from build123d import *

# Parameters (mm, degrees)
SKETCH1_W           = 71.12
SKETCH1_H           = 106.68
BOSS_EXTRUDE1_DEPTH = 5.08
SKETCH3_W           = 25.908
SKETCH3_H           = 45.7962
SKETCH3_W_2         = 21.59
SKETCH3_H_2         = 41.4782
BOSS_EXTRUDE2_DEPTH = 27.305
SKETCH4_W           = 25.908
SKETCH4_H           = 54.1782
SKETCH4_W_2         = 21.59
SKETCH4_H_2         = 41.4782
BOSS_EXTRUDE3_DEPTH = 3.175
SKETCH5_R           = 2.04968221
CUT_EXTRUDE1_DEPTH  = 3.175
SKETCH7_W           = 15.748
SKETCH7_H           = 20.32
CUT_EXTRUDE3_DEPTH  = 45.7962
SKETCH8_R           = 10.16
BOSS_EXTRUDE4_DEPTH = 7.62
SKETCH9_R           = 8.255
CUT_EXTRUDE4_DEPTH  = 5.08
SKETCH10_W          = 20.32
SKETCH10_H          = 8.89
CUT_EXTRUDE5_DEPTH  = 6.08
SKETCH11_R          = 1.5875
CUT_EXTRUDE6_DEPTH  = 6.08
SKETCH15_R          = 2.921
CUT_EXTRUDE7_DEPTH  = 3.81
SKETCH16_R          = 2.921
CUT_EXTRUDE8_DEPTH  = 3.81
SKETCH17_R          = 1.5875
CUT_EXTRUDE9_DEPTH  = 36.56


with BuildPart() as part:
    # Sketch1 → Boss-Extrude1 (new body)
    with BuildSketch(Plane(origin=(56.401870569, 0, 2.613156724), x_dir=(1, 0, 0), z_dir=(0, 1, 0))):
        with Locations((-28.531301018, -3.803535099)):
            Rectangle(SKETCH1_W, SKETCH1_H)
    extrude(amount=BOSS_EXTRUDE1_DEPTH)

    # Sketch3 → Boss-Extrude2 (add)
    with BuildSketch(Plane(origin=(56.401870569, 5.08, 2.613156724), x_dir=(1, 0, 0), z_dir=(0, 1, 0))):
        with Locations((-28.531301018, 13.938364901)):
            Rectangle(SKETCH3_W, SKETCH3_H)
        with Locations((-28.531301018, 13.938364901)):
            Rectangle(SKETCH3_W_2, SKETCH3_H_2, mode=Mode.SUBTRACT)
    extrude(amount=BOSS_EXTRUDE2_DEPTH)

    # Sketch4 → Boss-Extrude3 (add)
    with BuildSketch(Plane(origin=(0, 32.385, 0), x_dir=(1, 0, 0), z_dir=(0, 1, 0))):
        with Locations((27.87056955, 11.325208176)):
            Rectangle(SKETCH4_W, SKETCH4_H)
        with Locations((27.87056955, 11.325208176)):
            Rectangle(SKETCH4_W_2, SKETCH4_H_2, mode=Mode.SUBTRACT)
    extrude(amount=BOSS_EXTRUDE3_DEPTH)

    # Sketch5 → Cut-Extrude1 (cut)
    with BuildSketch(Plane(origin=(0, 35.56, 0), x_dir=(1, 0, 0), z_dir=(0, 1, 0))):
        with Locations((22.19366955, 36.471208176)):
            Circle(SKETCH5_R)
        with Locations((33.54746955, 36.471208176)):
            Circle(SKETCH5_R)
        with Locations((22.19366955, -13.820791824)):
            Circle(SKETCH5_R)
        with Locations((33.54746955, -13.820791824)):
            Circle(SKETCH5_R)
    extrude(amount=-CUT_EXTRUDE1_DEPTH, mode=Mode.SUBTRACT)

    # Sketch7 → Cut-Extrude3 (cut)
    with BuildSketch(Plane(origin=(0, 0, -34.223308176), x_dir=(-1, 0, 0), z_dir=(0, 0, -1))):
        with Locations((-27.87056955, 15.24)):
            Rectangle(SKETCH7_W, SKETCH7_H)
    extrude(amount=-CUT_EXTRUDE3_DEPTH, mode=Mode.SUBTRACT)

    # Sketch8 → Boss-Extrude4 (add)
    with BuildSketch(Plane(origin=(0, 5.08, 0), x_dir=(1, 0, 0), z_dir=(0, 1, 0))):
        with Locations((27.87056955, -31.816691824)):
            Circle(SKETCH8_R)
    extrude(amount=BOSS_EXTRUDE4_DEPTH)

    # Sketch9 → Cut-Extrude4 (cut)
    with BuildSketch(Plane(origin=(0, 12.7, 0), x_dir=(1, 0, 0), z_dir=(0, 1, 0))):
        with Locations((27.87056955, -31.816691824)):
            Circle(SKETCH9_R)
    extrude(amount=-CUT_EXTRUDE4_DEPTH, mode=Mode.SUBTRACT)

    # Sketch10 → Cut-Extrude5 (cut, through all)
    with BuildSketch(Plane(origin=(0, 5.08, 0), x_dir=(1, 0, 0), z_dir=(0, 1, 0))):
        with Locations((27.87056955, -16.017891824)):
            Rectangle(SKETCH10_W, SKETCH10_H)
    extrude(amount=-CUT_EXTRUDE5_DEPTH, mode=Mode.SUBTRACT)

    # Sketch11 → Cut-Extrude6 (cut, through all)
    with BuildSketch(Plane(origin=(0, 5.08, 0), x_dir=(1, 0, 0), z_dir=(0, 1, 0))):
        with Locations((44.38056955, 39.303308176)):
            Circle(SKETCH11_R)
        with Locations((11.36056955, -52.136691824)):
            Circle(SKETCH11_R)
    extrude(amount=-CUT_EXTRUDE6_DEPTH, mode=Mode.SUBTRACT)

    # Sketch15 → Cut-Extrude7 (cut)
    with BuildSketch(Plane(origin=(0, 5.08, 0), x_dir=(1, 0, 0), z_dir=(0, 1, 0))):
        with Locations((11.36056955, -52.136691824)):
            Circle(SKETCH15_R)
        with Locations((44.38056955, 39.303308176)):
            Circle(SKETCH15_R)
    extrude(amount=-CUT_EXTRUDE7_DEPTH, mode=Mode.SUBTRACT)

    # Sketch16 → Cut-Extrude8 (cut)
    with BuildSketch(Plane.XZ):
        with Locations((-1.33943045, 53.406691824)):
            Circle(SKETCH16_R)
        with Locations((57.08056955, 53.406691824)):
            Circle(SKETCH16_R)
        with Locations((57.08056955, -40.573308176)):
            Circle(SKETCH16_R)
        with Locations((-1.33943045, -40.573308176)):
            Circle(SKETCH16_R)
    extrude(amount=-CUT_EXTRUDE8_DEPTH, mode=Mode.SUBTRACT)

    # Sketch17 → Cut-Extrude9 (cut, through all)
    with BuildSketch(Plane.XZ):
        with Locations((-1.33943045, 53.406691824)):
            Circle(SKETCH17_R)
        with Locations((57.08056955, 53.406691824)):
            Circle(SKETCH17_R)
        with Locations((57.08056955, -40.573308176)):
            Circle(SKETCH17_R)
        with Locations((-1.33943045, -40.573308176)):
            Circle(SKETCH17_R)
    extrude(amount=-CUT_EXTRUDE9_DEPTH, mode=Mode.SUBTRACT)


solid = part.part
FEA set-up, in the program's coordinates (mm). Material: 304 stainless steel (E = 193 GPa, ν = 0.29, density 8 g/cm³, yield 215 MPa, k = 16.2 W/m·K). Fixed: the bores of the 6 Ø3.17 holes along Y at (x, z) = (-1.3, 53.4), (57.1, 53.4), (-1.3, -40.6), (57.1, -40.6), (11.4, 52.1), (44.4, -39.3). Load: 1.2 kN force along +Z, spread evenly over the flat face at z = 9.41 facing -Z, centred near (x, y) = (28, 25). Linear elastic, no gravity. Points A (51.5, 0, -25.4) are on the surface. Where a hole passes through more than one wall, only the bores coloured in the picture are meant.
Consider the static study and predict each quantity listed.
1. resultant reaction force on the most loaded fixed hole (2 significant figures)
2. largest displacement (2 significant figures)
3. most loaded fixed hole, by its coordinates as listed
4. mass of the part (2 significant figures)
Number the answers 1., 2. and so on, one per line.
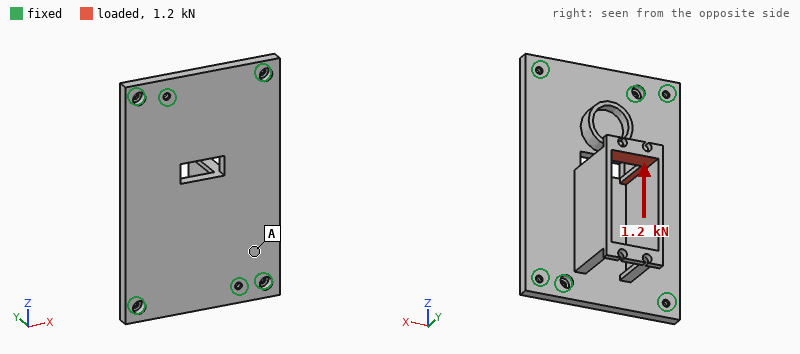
1. 850 N
2. 63 µm
3. (11.4, 52.1)
4. 370 g
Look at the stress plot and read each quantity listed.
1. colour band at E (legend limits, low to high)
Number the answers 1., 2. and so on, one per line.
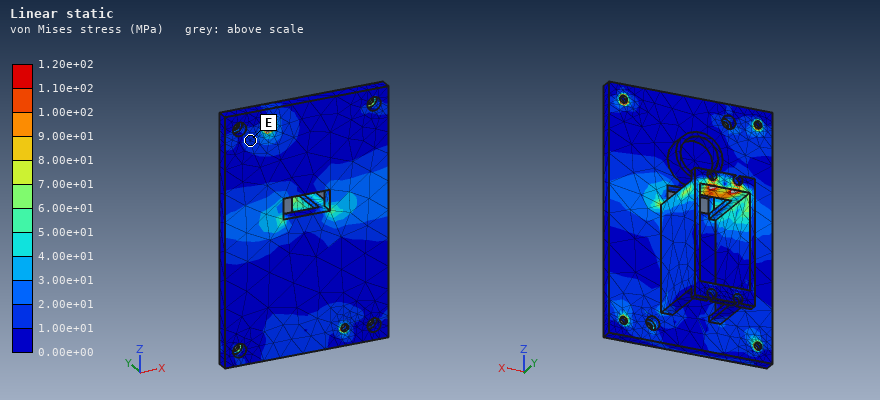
1. 1.00e+01 to 2.00e+01 MPa
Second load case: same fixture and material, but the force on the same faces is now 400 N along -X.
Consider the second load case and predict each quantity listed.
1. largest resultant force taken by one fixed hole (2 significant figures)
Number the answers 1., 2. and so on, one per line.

1. 150 N
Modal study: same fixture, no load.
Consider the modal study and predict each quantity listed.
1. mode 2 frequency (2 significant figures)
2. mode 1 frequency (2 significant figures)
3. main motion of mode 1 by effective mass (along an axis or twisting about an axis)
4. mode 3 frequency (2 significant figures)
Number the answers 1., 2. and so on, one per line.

1. 2600 Hz
2. 1800 Hz
3. along Y
4. 4200 Hz
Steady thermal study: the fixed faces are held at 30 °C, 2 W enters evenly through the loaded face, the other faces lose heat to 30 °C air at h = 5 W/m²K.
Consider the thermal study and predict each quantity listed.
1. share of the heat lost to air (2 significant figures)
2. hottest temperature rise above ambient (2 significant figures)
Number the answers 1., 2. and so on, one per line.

1. 40 %
2. 35 K
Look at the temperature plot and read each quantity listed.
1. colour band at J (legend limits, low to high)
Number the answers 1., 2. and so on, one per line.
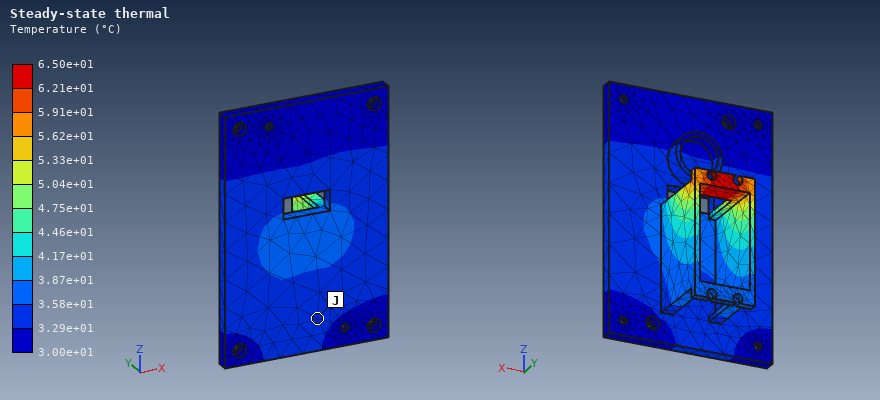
1. 3.29e+01 to 3.58e+01 °C
